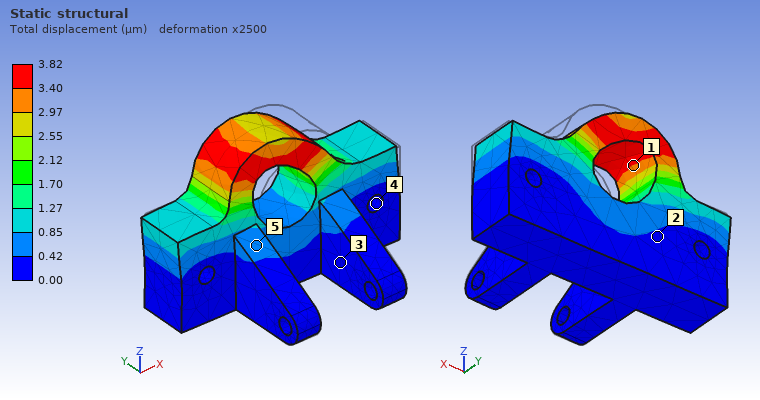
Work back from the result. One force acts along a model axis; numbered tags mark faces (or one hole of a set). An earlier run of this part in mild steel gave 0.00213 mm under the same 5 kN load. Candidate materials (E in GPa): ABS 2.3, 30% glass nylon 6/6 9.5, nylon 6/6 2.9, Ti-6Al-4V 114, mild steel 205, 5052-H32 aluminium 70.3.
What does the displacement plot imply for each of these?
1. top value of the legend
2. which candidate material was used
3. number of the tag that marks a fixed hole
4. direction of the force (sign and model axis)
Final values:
3.82 µm
Ti-6Al-4V
4
-X
